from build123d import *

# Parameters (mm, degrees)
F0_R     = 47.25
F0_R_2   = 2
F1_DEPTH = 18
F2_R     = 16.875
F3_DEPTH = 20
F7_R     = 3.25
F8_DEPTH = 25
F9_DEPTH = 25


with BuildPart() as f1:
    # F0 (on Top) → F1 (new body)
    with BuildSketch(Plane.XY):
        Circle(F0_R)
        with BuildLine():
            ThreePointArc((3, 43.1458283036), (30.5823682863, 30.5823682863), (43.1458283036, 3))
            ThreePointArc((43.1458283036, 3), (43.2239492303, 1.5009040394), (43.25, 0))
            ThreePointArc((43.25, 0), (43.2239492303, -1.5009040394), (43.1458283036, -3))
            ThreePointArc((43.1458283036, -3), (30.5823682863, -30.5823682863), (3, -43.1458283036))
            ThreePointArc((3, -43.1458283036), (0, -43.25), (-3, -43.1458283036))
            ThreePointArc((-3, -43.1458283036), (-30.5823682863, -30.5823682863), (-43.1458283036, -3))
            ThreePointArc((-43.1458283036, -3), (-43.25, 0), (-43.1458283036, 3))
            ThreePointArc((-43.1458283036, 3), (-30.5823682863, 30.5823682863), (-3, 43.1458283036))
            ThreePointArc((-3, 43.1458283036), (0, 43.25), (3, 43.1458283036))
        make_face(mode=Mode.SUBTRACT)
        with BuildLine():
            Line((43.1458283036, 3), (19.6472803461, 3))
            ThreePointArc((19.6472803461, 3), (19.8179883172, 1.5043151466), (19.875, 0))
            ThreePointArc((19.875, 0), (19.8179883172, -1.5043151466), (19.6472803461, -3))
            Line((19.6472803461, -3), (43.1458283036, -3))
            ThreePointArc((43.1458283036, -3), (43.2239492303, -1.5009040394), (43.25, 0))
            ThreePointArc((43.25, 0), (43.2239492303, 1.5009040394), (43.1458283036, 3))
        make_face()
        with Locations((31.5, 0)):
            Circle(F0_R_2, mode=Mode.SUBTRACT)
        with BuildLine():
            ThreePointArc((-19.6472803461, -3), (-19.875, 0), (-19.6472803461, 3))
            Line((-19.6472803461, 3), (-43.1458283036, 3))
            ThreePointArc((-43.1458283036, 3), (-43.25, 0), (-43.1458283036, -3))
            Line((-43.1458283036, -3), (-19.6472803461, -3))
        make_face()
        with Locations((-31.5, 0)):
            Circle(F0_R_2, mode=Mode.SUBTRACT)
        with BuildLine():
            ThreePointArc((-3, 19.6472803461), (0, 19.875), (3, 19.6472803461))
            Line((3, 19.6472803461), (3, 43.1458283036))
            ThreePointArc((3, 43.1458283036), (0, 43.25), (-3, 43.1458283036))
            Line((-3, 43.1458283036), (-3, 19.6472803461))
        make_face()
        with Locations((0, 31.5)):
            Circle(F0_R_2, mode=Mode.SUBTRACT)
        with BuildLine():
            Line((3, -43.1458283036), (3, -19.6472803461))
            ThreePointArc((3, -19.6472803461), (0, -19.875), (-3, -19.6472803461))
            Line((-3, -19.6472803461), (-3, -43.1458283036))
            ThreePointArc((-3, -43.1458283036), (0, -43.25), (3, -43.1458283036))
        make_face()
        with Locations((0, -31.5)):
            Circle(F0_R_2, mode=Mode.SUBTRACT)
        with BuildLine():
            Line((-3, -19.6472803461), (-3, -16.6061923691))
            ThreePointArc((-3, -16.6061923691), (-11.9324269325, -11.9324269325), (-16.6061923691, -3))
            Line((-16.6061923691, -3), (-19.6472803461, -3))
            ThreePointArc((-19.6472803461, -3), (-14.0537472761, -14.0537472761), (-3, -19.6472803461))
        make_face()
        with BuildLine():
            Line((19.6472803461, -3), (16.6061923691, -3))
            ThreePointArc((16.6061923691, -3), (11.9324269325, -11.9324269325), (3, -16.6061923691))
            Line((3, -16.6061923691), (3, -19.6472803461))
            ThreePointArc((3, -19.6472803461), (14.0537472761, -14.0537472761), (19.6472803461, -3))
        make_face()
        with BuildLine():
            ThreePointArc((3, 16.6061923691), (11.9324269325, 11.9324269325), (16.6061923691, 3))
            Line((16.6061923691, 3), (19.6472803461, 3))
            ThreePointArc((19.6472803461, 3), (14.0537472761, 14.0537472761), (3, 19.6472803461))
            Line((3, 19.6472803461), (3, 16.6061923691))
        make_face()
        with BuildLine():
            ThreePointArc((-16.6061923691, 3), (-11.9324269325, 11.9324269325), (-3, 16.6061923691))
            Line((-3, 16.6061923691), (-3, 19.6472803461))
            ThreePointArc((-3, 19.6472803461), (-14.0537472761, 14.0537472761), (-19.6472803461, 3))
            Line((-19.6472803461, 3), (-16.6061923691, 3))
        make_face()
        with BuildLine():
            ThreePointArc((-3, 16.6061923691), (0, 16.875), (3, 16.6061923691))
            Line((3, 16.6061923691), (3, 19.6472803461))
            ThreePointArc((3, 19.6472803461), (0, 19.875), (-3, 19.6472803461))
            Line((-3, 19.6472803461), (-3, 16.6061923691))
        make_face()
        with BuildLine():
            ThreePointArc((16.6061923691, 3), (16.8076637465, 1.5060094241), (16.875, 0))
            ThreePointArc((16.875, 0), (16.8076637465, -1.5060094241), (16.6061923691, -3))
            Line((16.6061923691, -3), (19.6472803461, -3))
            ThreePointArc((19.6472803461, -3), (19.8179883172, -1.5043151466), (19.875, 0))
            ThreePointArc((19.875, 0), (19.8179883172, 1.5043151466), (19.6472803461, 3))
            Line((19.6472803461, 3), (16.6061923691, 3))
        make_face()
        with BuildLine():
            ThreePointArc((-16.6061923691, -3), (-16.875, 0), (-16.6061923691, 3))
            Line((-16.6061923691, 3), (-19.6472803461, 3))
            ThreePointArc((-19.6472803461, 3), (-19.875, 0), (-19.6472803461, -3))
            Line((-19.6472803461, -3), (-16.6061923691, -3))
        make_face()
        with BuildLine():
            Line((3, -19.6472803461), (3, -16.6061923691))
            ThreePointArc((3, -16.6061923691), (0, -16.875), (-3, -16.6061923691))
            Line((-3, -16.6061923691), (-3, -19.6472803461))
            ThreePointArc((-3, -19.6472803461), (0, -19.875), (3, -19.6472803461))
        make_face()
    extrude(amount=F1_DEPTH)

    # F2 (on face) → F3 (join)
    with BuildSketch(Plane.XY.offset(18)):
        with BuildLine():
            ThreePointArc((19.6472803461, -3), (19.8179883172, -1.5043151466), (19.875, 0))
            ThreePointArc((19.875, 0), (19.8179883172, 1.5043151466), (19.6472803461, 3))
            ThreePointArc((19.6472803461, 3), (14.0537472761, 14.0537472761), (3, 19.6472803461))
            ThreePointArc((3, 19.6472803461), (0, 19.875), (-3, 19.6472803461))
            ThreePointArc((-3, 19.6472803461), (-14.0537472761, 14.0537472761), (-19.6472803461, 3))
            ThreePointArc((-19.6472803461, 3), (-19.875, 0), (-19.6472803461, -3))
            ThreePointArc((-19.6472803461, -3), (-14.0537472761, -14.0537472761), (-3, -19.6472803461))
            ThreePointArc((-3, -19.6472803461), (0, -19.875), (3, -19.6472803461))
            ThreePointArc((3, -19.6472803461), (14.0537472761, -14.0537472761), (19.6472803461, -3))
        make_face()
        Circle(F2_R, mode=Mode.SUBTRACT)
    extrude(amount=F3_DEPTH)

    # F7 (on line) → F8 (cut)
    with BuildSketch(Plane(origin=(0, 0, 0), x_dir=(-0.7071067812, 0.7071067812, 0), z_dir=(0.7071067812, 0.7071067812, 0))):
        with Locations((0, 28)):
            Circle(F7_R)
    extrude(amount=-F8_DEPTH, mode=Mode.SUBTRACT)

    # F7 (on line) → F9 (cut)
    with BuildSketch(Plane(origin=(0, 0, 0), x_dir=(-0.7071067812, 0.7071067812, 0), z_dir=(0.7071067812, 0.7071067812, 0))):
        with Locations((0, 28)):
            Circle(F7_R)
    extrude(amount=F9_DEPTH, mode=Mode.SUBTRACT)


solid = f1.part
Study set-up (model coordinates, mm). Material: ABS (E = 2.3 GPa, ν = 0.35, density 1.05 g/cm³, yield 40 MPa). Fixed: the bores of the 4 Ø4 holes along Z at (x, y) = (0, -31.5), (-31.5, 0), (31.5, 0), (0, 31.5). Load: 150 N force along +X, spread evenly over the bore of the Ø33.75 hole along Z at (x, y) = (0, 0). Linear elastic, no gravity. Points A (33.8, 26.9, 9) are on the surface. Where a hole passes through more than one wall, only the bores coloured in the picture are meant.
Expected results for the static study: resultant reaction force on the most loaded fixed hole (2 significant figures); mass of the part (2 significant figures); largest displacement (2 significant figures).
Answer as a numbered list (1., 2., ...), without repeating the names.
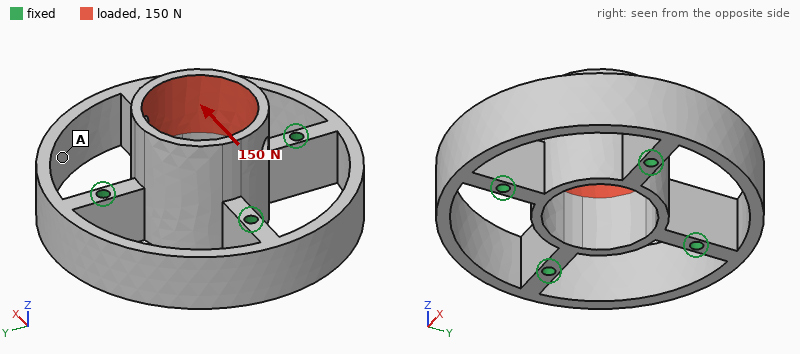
1. 73 N
2. 45 g
3. 56 µm
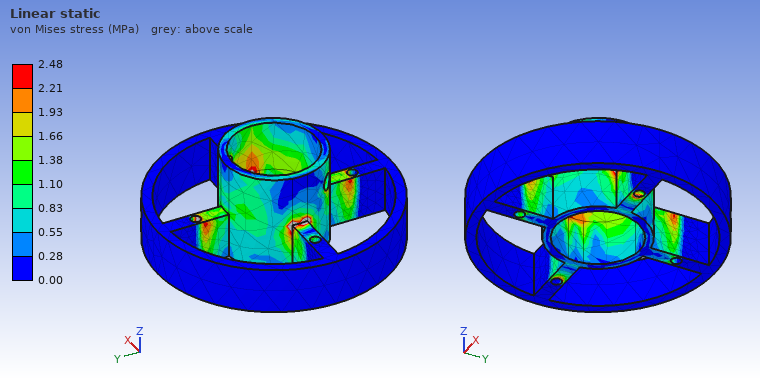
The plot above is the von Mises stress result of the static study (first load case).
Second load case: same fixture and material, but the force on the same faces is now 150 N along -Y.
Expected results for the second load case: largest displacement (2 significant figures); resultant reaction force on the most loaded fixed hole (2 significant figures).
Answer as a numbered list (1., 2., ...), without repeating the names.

1. 56 µm
2. 73 N
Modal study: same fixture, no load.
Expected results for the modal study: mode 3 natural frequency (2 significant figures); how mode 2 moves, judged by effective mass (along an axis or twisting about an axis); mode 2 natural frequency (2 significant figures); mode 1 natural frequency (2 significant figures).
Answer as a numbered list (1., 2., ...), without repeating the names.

1. 1900 Hz
2. twisting about Z
3. 1700 Hz
4. 1500 Hz
